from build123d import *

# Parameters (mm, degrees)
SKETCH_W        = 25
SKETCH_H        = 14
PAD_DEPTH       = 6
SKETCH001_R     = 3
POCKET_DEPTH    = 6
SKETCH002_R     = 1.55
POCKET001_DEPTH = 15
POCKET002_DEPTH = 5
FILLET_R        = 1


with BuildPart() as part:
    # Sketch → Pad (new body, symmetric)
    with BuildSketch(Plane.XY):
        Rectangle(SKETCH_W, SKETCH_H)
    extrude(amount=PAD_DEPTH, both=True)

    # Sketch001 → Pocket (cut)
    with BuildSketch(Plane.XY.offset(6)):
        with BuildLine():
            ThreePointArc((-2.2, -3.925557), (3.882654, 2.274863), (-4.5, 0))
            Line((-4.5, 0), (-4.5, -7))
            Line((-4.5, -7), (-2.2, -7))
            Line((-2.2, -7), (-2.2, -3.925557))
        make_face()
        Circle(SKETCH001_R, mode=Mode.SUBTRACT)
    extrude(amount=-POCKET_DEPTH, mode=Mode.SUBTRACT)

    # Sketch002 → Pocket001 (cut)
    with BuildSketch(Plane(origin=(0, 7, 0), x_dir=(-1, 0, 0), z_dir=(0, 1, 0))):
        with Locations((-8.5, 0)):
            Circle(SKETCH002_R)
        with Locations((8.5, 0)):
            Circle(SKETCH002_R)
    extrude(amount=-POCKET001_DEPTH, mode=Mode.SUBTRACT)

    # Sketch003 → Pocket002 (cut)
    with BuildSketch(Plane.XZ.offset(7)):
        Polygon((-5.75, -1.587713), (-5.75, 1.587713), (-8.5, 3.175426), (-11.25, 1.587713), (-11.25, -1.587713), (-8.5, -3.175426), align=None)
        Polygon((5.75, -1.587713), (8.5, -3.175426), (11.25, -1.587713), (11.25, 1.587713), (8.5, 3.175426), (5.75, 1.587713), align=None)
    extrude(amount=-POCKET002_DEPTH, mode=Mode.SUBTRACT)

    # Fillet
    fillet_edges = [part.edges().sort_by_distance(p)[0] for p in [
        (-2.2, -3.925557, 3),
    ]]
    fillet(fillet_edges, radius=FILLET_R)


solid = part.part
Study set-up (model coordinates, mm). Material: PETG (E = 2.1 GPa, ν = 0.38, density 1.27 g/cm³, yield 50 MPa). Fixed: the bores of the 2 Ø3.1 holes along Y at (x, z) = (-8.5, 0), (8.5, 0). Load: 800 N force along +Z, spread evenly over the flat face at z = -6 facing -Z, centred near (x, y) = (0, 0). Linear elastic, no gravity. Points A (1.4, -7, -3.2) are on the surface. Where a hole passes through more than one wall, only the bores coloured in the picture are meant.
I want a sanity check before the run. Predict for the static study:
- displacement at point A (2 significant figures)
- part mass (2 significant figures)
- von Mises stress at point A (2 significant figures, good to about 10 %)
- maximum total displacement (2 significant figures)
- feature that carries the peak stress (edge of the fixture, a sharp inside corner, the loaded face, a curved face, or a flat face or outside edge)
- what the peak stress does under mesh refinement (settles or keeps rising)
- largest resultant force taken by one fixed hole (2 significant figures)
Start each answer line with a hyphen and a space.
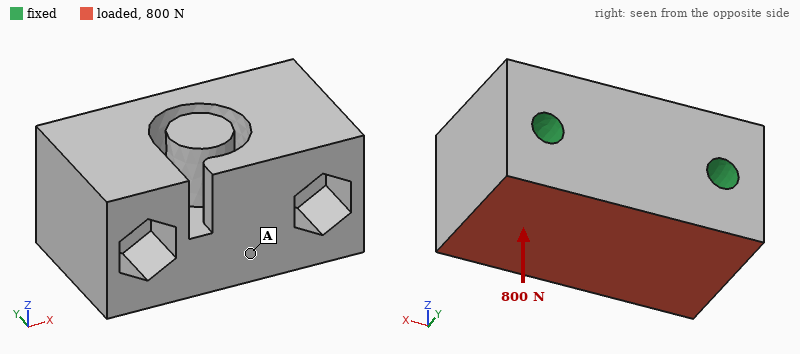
- 58 µm
- 4.5 g
- 2.8 MPa
- 66 µm
- edge of the fixture
- keeps rising
- 410 N
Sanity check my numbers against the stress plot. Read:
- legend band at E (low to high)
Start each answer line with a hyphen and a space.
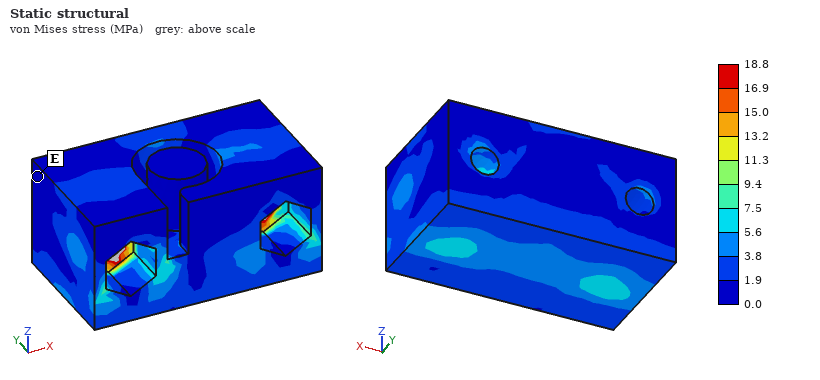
- 0.0 to 1.9 MPa
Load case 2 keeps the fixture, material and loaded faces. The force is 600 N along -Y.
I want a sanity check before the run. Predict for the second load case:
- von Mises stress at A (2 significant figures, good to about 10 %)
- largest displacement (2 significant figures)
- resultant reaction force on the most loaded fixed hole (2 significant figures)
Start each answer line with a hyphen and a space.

- 3.2 MPa
- 83 µm
- 300 N
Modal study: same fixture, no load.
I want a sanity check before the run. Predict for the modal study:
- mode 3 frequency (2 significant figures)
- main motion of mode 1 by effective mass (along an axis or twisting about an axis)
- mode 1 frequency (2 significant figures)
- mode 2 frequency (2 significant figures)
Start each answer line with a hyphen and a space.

- 14 kHz
- along Z
- 10 kHz
- 12 kHz
